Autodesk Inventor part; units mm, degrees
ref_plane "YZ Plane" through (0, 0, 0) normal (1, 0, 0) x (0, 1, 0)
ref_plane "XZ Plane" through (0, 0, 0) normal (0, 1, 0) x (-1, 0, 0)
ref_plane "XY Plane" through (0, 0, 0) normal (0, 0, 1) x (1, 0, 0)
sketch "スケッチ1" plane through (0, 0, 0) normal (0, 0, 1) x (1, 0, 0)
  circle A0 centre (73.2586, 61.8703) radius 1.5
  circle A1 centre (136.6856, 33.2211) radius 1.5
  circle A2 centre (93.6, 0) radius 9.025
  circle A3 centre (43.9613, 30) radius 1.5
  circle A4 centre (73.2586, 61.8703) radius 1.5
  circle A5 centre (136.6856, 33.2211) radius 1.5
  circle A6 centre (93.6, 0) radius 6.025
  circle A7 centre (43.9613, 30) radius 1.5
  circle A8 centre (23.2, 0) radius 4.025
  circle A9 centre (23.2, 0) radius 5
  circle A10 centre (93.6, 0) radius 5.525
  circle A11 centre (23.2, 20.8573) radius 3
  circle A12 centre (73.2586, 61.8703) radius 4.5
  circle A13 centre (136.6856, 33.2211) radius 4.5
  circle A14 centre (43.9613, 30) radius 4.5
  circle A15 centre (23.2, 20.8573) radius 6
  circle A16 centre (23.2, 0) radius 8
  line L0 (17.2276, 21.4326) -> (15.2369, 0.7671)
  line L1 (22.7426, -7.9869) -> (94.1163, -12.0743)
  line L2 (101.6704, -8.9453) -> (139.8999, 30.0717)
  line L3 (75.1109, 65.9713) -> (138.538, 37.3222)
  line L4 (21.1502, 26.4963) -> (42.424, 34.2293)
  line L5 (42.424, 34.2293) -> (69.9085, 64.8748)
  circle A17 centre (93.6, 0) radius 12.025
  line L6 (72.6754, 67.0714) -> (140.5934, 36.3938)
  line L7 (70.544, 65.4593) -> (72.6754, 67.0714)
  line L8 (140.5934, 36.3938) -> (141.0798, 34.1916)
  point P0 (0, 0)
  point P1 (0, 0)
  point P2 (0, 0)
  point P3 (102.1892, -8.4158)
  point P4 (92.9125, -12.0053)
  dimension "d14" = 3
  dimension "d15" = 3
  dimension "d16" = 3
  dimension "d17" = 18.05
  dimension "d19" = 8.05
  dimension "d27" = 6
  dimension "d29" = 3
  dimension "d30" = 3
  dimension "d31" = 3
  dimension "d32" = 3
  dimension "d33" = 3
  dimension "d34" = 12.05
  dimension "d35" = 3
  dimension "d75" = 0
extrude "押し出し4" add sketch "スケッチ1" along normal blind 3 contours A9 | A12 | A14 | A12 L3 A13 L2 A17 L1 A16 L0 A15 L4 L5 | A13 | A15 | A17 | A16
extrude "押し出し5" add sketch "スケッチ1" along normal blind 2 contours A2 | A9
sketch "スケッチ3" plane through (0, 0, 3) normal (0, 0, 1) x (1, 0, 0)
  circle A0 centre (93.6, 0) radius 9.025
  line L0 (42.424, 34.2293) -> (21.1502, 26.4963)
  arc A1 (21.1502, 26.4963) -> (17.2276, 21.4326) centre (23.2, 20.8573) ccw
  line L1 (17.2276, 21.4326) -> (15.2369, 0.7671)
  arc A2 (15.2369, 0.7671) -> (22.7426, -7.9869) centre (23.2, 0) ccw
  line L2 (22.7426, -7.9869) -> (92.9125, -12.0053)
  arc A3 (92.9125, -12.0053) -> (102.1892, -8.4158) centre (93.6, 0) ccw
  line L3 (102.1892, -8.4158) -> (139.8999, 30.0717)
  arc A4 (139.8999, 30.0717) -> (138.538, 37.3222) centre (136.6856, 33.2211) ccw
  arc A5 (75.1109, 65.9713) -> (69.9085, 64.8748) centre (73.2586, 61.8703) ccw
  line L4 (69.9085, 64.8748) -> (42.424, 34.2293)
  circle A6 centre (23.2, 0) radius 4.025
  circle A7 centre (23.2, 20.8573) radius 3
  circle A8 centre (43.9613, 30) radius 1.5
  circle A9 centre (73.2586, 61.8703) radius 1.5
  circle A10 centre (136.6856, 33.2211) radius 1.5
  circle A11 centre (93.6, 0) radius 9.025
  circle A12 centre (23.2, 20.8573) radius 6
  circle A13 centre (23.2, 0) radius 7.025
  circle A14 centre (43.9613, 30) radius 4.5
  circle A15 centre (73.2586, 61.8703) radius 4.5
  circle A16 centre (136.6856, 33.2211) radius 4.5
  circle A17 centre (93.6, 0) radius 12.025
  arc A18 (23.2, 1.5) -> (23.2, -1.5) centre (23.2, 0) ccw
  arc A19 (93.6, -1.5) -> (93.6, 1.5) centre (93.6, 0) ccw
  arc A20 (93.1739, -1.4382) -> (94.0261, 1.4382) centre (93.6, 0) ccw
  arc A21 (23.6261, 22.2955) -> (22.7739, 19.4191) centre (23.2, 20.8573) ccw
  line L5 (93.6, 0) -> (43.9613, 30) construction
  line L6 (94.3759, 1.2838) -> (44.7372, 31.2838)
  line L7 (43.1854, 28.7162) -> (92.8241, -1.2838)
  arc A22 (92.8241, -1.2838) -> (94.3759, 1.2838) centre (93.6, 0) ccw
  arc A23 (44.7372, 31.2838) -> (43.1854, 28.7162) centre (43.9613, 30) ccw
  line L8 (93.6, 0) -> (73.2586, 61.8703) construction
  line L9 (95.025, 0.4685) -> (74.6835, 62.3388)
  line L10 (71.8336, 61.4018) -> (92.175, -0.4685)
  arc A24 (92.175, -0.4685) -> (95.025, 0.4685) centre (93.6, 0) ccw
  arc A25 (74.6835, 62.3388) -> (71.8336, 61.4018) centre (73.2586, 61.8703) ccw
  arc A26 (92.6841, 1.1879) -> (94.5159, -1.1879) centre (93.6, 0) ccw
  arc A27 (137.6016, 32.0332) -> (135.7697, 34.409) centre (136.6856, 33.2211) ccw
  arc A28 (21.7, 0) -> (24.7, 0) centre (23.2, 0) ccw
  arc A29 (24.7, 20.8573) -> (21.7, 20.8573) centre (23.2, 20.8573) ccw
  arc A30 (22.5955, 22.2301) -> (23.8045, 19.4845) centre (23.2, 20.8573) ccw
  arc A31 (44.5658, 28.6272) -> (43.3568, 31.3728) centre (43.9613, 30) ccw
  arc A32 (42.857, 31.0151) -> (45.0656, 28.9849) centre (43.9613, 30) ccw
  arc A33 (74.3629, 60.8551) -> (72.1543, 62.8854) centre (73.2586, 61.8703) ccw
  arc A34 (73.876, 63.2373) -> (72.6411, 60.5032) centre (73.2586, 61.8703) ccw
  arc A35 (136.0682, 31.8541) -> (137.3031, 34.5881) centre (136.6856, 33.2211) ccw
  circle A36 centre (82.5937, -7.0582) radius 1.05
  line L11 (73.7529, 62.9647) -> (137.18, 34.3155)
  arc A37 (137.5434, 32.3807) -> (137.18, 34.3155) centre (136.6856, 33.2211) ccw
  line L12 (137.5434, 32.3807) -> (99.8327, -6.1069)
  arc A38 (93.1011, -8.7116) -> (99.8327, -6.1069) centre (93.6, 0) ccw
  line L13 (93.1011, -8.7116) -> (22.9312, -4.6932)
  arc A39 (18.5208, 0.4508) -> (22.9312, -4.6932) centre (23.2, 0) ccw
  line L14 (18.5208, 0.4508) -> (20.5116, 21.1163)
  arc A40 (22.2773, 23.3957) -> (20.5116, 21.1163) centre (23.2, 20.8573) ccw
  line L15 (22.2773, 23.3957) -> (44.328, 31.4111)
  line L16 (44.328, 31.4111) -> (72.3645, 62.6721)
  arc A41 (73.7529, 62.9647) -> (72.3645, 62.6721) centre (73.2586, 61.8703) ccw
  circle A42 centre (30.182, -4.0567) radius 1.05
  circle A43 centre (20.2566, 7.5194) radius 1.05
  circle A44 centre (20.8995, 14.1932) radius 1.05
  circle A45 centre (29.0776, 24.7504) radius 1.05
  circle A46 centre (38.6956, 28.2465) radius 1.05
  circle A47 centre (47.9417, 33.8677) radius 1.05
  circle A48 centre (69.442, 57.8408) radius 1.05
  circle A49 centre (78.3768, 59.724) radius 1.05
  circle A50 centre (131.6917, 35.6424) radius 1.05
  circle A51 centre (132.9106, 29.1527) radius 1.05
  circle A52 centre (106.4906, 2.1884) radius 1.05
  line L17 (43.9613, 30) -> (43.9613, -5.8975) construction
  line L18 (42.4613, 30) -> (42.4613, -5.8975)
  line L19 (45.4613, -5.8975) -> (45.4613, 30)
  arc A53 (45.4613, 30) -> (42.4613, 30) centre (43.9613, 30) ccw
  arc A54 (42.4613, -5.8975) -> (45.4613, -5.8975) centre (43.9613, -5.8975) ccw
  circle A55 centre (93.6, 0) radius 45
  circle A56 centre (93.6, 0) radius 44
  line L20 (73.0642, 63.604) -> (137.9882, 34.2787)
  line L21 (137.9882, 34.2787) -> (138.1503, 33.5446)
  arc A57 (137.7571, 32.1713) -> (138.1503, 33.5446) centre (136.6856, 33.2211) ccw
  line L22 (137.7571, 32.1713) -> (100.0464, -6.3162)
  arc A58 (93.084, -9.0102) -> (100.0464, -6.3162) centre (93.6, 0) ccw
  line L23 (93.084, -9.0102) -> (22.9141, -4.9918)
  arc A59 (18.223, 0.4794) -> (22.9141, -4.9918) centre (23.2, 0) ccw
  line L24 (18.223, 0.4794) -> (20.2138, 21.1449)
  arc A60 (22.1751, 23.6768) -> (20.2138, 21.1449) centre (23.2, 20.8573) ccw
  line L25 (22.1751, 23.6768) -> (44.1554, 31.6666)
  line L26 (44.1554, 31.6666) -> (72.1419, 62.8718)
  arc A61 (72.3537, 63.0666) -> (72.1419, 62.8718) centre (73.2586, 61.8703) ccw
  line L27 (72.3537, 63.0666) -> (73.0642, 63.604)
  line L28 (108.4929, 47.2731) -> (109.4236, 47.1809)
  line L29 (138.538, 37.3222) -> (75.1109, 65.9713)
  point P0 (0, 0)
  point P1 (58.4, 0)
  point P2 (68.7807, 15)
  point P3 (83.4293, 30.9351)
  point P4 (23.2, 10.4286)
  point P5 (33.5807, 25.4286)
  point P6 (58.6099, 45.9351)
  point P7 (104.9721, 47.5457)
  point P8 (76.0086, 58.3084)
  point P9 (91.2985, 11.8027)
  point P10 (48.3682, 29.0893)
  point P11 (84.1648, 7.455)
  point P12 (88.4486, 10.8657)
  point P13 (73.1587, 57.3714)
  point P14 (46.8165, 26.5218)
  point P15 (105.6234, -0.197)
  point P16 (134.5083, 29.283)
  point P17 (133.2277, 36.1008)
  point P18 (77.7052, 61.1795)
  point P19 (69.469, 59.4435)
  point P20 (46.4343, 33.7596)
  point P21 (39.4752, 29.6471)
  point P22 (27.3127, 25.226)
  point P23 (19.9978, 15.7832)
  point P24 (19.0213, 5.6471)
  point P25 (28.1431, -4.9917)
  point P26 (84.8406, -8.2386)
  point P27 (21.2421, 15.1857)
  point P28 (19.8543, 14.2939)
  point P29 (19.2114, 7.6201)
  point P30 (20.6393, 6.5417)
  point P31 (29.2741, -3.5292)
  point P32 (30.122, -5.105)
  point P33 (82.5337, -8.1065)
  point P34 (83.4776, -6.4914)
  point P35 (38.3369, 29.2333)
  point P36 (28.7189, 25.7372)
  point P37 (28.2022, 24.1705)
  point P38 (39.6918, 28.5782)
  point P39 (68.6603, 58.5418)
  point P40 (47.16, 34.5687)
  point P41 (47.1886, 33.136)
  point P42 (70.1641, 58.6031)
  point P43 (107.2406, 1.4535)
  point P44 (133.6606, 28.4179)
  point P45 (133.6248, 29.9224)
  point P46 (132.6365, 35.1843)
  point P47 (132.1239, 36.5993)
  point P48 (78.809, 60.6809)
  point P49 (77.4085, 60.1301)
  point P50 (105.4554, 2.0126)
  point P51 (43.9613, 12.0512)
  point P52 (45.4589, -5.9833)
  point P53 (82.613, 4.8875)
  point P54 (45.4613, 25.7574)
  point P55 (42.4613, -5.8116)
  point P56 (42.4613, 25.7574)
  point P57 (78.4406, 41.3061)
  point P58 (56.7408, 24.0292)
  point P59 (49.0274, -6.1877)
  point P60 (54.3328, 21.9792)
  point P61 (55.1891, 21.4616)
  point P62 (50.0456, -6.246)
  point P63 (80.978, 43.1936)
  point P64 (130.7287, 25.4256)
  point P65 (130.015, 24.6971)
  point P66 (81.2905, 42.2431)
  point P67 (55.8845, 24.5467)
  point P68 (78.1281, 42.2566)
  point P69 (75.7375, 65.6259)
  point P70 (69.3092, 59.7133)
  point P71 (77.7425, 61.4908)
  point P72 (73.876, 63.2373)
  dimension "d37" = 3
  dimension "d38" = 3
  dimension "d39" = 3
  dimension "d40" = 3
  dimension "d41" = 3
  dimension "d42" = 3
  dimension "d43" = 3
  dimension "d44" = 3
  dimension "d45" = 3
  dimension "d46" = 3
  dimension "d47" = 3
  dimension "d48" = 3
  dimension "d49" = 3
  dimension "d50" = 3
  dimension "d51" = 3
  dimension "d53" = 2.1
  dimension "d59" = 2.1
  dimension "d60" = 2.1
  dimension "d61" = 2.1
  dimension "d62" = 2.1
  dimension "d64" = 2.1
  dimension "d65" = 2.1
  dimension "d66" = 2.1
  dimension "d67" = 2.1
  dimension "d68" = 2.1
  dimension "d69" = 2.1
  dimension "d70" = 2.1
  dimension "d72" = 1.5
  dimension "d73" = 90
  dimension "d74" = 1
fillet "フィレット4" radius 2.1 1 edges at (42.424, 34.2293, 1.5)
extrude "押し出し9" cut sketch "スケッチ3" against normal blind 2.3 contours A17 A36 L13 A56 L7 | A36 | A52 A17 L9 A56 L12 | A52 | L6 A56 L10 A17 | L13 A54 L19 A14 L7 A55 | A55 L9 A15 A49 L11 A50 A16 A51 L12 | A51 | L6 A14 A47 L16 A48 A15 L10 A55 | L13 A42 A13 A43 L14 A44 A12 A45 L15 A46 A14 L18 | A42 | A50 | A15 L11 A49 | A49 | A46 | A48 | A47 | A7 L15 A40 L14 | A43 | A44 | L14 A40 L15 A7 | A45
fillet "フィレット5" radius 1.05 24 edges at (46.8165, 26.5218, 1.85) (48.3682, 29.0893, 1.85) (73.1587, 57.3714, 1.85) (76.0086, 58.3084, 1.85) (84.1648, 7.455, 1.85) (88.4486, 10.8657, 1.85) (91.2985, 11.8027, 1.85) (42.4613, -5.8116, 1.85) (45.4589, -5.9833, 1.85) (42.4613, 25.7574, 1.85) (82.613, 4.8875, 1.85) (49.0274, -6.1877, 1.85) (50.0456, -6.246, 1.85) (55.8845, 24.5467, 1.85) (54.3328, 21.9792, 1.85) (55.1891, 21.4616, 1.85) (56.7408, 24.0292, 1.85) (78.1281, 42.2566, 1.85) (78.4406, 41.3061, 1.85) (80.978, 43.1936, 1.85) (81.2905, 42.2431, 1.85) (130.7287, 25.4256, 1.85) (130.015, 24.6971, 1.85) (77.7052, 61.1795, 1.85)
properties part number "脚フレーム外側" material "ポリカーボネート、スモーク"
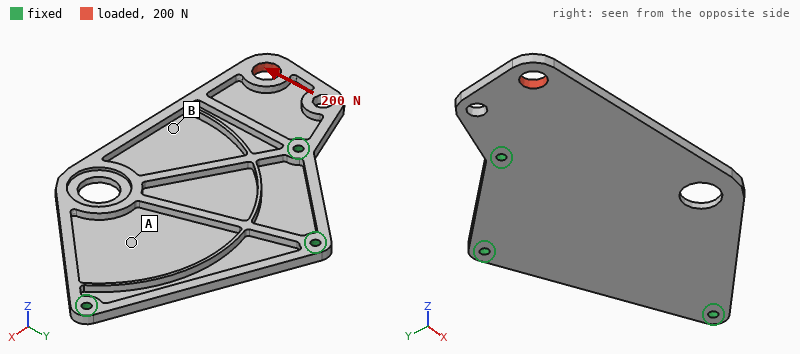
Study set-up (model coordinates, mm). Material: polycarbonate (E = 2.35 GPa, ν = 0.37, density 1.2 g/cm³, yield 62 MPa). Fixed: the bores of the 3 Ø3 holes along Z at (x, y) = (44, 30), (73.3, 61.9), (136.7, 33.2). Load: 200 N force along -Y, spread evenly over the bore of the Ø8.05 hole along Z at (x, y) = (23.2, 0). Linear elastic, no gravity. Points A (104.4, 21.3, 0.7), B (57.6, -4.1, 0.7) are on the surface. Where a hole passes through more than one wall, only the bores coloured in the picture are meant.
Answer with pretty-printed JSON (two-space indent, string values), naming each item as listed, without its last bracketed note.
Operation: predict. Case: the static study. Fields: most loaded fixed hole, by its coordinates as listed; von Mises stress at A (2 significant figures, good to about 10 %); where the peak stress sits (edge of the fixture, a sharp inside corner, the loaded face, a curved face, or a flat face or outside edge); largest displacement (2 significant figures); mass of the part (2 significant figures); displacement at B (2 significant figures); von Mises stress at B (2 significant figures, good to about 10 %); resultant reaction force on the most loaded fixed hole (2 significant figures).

{
  "most loaded fixed hole, by its coordinates as listed": "(44, 30)",
  "von Mises stress at A": "2.2 MPa",
  "where the peak stress sits": "a curved face",
  "largest displacement": "1.6 mm",
  "mass of the part": "10 g",
  "displacement at B": "0.26 mm",
  "von Mises stress at B": "5.7 MPa",
  "resultant reaction force on the most loaded fixed hole": "250 N"
}
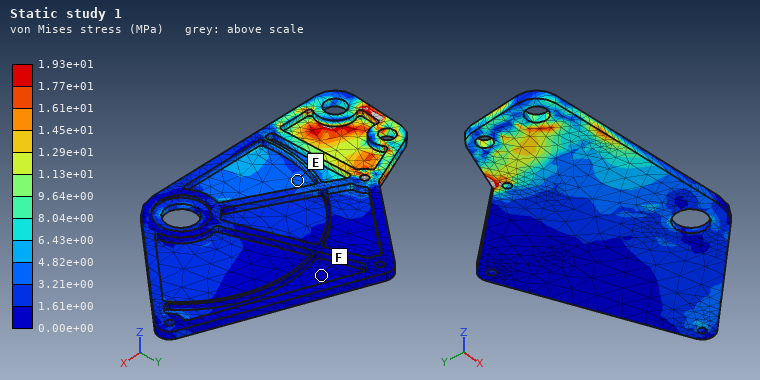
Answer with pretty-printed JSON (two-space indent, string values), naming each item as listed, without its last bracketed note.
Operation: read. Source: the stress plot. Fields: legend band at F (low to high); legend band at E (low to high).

{
  "legend band at F": "0.00e+00 to 1.61e+00 MPa",
  "legend band at E": "3.21e+00 to 4.82e+00 MPa"
}
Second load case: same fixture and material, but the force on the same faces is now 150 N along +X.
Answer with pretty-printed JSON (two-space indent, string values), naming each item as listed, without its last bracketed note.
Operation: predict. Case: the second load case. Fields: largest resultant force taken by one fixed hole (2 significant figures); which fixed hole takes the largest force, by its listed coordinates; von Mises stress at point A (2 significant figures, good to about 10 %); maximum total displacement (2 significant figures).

{
  "largest resultant force taken by one fixed hole": "110 N",
  "which fixed hole takes the largest force, by its listed coordinates": "(44, 30)",
  "von Mises stress at point A": "2.6 MPa",
  "maximum total displacement": "1.6 mm"
}
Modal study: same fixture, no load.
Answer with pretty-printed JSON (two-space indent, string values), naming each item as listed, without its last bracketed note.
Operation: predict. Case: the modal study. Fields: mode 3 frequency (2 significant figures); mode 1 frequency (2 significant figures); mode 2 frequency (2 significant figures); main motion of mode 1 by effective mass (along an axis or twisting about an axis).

{
  "mode 3 frequency": "580 Hz",
  "mode 1 frequency": "210 Hz",
  "mode 2 frequency": "290 Hz",
  "main motion of mode 1 by effective mass": "along Z"
}
